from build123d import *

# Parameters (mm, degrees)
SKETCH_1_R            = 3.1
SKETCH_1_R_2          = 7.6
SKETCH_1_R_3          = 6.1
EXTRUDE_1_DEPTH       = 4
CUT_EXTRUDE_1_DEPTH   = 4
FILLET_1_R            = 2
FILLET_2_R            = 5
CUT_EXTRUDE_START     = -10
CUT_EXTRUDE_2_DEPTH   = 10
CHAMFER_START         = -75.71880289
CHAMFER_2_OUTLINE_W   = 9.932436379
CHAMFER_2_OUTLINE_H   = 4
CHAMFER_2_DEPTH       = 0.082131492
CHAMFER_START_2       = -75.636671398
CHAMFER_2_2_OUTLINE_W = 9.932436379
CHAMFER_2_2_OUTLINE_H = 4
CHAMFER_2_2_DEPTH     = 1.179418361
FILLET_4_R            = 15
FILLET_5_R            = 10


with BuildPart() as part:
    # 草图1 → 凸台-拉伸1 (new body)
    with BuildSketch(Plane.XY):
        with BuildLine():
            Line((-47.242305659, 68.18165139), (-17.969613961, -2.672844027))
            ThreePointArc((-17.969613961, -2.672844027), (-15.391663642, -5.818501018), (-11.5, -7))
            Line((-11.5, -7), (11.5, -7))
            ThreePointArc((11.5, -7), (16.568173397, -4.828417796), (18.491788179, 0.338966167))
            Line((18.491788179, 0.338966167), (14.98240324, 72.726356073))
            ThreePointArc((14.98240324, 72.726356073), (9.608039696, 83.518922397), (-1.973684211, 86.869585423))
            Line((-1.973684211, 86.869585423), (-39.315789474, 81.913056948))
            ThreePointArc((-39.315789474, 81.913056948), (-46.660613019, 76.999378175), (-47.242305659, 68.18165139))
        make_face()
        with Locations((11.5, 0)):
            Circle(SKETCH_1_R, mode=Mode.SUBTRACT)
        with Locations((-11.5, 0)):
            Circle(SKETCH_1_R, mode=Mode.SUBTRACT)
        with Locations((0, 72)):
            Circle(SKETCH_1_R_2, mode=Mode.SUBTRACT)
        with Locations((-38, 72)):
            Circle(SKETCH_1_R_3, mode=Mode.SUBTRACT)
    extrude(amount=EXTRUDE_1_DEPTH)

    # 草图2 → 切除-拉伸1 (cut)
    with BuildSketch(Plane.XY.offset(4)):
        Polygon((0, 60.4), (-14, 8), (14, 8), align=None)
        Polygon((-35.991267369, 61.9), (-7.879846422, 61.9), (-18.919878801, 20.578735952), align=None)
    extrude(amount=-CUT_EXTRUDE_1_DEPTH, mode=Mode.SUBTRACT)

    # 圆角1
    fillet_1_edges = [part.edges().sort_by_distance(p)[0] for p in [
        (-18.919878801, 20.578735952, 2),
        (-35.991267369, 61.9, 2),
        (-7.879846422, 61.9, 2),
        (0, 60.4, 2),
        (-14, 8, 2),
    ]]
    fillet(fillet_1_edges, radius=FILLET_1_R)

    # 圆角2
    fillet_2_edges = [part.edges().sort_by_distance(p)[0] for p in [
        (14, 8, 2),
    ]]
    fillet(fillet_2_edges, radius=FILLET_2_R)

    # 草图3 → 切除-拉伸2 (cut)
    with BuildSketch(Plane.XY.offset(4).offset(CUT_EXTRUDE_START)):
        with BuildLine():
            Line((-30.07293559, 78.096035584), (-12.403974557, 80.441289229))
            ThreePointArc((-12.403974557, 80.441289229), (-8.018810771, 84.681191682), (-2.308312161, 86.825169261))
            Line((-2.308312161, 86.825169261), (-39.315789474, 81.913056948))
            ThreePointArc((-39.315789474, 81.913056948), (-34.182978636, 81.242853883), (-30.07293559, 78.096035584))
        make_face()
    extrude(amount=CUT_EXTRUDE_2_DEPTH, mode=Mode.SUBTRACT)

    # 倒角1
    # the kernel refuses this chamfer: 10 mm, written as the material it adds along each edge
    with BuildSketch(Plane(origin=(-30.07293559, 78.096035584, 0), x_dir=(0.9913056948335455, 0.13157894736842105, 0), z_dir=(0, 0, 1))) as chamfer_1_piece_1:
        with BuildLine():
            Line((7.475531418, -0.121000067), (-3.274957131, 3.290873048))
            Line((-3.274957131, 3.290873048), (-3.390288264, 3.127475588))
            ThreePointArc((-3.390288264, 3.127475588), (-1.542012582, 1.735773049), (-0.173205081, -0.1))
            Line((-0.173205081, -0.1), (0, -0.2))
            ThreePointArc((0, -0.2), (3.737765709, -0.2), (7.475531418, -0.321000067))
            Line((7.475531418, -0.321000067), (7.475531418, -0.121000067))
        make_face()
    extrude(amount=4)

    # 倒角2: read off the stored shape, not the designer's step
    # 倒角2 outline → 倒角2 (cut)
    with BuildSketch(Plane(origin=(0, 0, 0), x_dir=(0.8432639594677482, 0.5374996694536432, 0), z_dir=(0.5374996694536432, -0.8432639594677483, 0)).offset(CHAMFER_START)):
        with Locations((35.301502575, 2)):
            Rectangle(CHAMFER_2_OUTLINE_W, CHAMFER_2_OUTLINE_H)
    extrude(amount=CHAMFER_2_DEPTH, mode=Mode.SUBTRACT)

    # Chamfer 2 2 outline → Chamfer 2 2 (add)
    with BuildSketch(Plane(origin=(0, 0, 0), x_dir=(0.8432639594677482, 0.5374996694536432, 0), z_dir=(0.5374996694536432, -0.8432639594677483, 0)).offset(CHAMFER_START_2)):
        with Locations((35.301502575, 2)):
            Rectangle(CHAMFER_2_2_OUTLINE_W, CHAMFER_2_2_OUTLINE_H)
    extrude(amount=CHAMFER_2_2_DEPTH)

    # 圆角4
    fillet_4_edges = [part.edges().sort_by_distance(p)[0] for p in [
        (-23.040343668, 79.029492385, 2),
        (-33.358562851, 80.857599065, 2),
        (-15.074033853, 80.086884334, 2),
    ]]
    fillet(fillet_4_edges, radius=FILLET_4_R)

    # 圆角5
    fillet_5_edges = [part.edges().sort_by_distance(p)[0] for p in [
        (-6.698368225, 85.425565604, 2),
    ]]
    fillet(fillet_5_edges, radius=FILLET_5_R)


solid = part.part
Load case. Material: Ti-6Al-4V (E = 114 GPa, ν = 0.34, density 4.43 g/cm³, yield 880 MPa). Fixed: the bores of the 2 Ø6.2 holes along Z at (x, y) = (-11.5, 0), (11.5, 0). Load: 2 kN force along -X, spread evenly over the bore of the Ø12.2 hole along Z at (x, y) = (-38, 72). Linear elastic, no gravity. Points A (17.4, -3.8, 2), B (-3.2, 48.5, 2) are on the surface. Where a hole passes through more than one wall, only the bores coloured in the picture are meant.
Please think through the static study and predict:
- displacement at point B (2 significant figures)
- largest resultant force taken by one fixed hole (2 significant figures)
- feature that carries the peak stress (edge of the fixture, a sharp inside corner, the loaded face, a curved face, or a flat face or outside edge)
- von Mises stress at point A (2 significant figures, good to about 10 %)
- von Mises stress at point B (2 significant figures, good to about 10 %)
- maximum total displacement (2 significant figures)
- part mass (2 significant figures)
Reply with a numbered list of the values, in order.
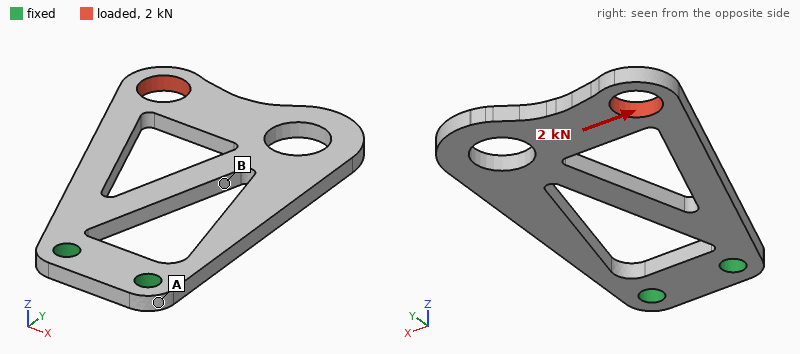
1. 0.26 mm
2. 4.5 kN
3. a curved face
4. 57 MPa
5. 200 MPa
6. 0.44 mm
7. 51 g
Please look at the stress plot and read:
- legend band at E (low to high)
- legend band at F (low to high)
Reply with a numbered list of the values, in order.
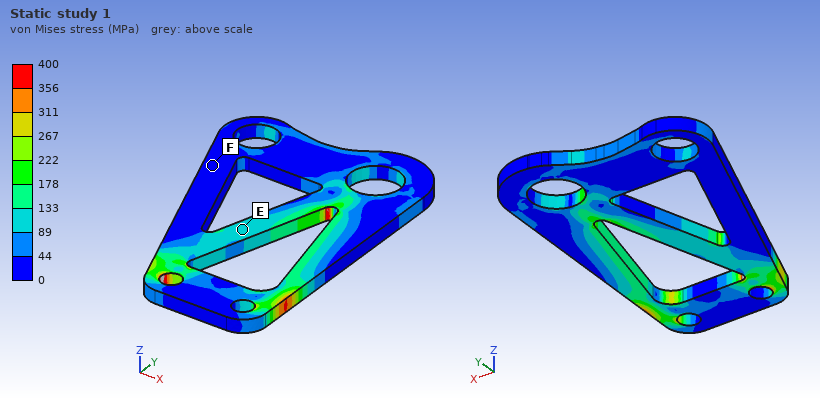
1. 89 to 133 MPa
2. 0 to 44 MPa
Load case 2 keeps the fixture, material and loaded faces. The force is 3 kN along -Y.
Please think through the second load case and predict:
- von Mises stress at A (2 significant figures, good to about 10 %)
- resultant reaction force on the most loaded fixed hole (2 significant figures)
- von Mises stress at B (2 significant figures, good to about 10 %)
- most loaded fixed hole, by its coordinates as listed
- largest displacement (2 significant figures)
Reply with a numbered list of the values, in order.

1. 27 MPa
2. 5.2 kN
3. 84 MPa
4. (-11.5, 0)
5. 0.30 mm
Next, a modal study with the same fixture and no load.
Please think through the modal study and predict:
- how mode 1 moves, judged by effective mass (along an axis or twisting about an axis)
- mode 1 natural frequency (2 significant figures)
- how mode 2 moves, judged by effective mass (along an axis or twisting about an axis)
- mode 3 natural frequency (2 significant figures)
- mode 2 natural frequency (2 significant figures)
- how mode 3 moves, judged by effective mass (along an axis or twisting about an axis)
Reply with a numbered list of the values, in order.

1. along Z
2. 340 Hz
3. twisting about Y
4. 2300 Hz
5. 970 Hz
6. along X
